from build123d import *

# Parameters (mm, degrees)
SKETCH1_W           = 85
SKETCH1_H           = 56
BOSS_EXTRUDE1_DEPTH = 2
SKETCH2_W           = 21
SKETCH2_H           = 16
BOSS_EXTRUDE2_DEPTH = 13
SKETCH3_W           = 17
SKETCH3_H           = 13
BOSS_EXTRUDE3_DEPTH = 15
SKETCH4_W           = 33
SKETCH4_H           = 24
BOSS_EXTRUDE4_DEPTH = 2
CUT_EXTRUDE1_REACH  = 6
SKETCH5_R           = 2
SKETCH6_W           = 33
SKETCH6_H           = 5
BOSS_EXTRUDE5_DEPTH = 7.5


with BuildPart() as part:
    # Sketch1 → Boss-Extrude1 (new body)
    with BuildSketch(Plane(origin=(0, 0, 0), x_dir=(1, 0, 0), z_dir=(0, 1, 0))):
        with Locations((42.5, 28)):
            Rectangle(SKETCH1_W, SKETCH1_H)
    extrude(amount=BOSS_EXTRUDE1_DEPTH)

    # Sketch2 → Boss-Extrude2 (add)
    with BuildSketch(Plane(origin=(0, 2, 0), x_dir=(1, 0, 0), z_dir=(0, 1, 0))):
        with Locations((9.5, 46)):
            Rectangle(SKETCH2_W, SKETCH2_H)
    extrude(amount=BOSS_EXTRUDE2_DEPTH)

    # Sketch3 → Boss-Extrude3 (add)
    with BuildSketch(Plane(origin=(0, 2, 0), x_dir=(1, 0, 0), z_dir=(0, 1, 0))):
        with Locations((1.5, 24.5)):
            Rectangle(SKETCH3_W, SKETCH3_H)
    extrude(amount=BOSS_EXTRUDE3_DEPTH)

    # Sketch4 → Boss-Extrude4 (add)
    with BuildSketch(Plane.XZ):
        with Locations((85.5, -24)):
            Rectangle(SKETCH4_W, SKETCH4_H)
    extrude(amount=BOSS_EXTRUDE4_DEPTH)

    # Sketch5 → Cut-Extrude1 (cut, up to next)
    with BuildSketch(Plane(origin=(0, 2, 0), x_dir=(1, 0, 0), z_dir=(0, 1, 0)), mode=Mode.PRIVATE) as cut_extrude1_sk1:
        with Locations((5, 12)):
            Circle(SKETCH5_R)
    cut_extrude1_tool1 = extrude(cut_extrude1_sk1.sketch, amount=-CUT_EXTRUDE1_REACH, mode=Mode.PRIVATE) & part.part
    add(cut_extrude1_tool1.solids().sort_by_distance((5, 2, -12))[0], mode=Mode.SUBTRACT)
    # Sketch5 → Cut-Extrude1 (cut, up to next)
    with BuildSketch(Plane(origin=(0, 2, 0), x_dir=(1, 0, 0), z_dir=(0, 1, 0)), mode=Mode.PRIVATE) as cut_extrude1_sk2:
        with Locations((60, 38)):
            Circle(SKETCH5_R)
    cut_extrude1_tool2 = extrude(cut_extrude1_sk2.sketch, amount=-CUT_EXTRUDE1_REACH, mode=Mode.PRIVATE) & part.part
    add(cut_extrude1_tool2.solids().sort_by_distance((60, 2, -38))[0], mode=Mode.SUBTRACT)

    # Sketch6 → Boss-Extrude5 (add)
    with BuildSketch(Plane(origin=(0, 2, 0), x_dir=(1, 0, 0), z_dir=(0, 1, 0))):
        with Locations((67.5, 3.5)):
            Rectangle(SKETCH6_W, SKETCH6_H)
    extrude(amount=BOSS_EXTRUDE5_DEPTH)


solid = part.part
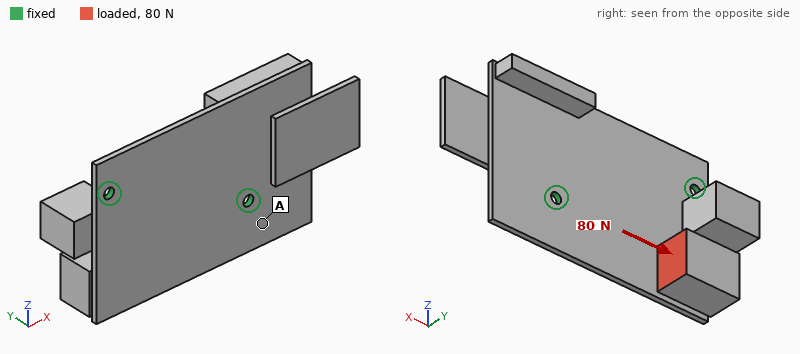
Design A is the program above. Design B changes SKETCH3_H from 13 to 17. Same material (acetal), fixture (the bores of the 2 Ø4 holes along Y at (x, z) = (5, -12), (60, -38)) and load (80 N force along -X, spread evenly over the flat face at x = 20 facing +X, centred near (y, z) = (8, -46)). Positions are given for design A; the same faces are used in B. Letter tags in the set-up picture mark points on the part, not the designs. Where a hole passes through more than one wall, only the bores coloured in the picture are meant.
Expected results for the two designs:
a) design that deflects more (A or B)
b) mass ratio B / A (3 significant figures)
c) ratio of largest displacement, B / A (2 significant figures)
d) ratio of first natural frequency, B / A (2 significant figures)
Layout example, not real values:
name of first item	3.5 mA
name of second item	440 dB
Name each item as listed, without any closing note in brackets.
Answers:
design that deflects more	A
mass ratio B / A	1.05
ratio of largest displacement, B / A	0.73
ratio of first natural frequency, B / A	1.1
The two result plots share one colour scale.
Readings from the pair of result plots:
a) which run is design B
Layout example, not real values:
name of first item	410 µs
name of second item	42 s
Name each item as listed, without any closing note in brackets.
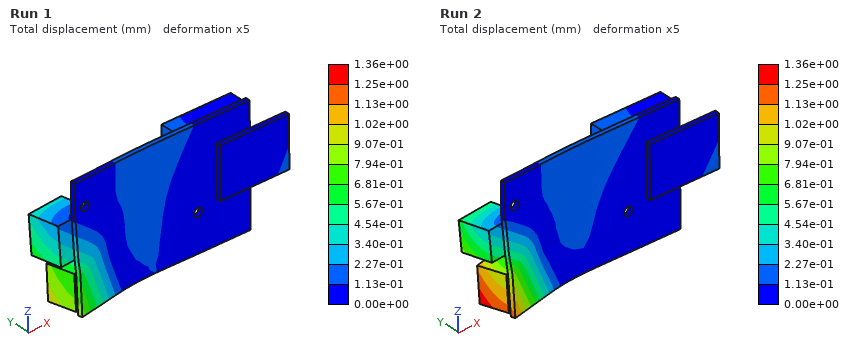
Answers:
which run is design B	Run 1
